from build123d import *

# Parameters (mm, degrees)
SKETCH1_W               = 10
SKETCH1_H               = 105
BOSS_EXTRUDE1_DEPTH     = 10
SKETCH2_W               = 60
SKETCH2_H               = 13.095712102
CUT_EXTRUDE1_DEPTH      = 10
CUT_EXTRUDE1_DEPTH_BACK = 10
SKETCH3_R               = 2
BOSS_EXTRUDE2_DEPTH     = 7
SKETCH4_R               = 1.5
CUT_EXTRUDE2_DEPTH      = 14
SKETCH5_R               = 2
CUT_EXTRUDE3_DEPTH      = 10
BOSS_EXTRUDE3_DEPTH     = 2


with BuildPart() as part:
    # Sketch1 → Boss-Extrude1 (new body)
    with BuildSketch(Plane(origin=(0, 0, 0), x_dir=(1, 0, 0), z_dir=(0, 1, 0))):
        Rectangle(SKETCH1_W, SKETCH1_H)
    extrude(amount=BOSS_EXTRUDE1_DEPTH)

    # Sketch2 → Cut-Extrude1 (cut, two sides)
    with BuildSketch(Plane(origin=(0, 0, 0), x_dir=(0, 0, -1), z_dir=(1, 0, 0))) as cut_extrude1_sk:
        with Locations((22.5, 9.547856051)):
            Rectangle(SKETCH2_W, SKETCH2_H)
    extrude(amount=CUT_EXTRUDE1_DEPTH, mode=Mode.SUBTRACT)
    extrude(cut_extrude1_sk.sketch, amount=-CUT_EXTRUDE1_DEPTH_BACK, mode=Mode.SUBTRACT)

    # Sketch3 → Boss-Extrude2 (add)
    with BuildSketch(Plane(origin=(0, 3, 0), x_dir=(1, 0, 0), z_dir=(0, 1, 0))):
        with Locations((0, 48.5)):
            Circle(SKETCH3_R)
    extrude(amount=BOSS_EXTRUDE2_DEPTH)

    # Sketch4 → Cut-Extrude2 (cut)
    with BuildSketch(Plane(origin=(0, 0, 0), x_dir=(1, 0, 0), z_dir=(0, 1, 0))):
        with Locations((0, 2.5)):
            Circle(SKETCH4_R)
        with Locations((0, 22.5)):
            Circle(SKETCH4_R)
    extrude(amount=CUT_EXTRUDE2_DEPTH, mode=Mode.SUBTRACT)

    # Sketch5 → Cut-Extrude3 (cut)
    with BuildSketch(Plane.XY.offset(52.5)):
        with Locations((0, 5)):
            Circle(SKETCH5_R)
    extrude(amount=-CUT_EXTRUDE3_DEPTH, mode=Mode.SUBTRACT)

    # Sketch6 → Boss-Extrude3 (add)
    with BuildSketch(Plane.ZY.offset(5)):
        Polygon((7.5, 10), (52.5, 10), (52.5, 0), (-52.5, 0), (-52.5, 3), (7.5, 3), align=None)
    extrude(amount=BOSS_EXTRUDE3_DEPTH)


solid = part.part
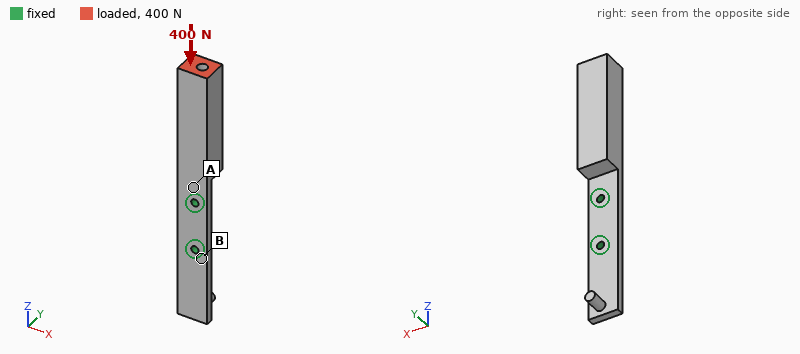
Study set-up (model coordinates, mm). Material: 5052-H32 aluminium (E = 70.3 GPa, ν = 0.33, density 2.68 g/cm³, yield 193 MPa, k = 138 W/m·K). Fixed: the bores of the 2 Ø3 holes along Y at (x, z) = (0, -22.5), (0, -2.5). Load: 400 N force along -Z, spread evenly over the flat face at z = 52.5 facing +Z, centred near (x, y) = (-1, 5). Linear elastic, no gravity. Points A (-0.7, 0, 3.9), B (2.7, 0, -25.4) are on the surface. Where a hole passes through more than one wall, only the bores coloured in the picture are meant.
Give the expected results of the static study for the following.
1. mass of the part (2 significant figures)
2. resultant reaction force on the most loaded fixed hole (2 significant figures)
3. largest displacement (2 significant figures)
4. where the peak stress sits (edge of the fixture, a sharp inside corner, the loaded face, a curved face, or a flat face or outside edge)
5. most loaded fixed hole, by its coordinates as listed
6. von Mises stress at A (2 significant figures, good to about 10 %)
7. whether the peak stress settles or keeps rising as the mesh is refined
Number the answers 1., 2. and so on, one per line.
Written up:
1. 20 g
2. 360 N
3. 0.40 mm
4. edge of the fixture
5. (0, -2.5)
6. 59 MPa
7. keeps rising
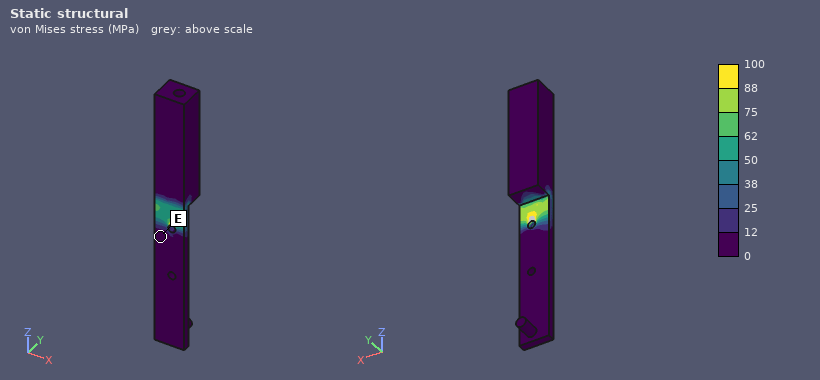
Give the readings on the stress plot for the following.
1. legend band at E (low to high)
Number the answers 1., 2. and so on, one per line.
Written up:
1. 0 to 12 MPa
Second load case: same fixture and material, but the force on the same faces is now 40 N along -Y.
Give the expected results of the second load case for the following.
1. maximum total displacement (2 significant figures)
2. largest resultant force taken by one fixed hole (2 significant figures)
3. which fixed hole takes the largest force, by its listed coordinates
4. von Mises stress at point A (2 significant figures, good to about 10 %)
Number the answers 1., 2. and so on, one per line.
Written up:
1. 0.58 mm
2. 53 N
3. (0, -2.5)
4. 99 MPa
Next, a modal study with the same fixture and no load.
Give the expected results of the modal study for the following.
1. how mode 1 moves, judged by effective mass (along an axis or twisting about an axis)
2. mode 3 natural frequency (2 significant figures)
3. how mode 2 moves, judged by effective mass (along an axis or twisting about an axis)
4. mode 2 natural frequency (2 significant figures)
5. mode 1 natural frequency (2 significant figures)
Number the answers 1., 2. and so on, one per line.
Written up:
1. along Y
2. 2500 Hz
3. along X
4. 1700 Hz
5. 590 Hz
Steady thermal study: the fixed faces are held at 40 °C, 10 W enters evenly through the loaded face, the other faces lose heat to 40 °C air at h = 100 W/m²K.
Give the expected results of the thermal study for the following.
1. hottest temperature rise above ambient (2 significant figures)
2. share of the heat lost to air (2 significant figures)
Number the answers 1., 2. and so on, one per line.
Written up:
1. 33 K
2. 49 %
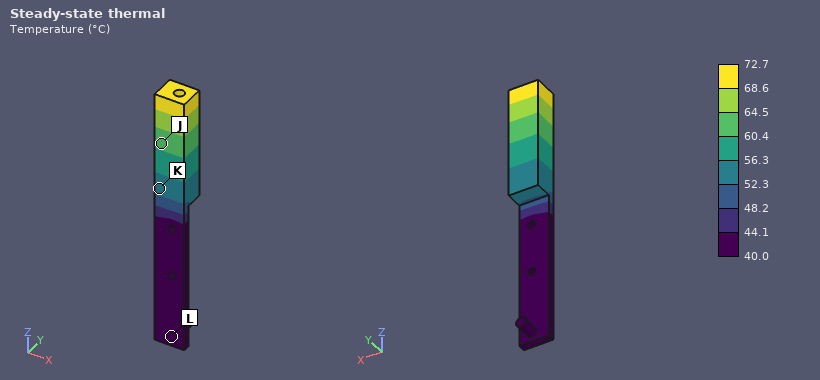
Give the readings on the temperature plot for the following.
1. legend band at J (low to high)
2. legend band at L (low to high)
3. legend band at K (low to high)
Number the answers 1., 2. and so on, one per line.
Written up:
1. 60.4 to 64.5 °C
2. 40.0 to 44.1 °C
3. 52.3 to 56.3 °C
